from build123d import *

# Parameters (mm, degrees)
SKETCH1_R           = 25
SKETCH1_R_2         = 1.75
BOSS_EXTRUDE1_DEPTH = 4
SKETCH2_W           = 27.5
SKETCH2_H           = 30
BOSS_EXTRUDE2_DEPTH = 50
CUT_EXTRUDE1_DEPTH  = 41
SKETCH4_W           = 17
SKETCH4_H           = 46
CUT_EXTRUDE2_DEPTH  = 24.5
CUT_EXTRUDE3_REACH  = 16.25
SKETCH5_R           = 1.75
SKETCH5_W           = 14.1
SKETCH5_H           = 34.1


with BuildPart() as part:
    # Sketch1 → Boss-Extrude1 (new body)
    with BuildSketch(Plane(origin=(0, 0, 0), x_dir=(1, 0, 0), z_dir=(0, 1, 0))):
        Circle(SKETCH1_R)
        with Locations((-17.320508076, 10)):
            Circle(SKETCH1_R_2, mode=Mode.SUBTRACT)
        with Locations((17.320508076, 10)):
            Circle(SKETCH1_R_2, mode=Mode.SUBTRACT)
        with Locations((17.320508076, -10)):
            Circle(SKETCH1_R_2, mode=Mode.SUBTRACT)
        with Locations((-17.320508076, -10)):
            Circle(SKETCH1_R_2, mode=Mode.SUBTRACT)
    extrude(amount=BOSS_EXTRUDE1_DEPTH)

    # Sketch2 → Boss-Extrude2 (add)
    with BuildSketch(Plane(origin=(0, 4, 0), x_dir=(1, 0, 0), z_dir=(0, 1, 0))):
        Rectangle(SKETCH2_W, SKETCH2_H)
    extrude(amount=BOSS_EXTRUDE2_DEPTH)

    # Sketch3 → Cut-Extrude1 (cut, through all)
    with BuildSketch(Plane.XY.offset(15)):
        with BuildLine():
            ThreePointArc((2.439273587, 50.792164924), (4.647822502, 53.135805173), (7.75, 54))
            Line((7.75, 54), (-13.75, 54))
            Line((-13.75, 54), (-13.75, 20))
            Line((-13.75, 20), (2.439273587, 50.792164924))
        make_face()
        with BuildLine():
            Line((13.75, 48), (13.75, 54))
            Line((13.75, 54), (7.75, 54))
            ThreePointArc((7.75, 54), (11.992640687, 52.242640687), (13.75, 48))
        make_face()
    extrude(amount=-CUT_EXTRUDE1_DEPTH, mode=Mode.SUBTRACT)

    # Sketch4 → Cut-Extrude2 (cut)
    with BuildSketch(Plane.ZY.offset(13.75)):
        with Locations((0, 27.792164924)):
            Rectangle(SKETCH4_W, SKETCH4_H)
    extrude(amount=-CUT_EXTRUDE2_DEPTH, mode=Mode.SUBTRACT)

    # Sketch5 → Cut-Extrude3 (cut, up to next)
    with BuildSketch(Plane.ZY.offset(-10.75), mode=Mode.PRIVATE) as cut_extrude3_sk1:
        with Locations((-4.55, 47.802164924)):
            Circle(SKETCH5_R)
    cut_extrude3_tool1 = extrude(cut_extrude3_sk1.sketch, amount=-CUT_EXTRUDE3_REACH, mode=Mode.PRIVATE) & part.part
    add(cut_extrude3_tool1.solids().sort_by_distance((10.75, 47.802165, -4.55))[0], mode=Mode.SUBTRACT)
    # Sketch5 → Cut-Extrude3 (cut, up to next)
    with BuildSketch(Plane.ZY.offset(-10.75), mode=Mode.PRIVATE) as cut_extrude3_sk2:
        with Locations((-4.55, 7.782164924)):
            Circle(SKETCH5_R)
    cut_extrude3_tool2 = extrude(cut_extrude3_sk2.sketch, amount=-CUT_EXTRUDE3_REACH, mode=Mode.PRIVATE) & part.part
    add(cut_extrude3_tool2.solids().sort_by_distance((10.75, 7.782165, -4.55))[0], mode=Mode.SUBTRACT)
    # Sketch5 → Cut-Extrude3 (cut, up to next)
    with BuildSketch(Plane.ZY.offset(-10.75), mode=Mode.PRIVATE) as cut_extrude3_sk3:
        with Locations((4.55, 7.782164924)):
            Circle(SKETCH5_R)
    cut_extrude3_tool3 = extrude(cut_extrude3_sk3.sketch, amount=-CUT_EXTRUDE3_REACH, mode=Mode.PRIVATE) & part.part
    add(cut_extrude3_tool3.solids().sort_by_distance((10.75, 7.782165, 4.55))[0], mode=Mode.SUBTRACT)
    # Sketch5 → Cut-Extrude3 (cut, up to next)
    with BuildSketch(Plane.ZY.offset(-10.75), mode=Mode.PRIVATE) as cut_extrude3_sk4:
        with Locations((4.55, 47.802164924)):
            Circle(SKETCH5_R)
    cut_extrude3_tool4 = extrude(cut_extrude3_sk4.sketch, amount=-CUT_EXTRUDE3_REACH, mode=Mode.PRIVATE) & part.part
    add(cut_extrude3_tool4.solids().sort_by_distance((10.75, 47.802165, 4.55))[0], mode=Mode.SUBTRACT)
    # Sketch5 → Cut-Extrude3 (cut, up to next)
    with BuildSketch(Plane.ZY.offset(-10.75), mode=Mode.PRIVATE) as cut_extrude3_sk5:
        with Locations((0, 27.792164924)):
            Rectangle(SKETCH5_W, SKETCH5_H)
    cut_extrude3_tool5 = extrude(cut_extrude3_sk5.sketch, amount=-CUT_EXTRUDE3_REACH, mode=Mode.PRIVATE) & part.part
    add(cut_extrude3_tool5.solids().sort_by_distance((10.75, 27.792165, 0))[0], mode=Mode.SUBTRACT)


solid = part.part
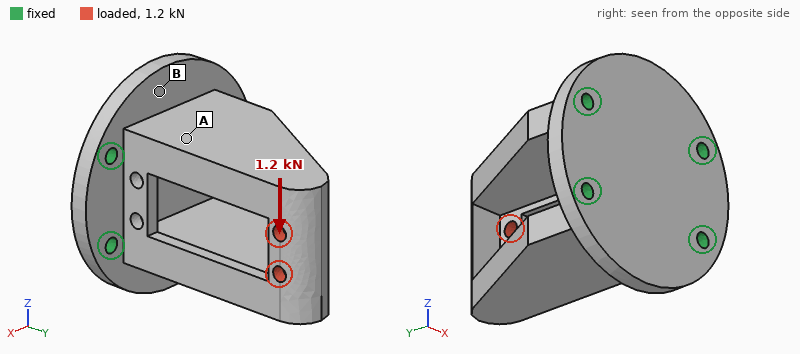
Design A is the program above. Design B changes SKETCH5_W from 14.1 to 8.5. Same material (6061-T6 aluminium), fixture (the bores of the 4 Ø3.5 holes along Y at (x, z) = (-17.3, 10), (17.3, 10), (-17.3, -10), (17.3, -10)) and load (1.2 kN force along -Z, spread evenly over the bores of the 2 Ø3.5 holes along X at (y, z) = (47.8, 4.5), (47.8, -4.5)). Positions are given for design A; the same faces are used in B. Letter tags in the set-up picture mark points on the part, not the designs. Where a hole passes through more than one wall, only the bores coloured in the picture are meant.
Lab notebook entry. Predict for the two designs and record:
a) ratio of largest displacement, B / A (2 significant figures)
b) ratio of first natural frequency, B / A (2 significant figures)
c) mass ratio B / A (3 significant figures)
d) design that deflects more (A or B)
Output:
0.75
1.1
1.02
A
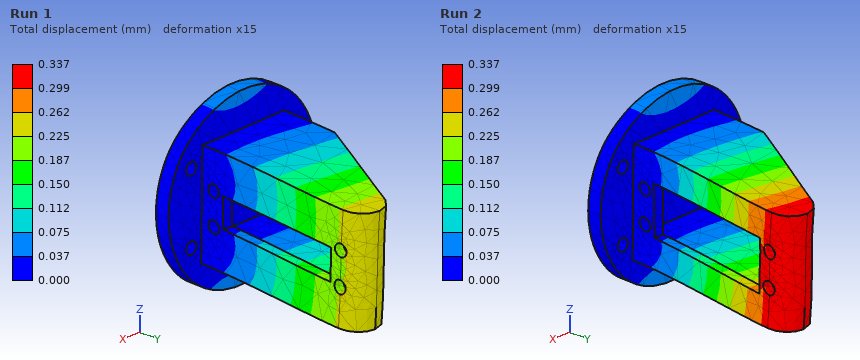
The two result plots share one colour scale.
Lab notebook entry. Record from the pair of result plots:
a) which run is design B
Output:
Run 1
